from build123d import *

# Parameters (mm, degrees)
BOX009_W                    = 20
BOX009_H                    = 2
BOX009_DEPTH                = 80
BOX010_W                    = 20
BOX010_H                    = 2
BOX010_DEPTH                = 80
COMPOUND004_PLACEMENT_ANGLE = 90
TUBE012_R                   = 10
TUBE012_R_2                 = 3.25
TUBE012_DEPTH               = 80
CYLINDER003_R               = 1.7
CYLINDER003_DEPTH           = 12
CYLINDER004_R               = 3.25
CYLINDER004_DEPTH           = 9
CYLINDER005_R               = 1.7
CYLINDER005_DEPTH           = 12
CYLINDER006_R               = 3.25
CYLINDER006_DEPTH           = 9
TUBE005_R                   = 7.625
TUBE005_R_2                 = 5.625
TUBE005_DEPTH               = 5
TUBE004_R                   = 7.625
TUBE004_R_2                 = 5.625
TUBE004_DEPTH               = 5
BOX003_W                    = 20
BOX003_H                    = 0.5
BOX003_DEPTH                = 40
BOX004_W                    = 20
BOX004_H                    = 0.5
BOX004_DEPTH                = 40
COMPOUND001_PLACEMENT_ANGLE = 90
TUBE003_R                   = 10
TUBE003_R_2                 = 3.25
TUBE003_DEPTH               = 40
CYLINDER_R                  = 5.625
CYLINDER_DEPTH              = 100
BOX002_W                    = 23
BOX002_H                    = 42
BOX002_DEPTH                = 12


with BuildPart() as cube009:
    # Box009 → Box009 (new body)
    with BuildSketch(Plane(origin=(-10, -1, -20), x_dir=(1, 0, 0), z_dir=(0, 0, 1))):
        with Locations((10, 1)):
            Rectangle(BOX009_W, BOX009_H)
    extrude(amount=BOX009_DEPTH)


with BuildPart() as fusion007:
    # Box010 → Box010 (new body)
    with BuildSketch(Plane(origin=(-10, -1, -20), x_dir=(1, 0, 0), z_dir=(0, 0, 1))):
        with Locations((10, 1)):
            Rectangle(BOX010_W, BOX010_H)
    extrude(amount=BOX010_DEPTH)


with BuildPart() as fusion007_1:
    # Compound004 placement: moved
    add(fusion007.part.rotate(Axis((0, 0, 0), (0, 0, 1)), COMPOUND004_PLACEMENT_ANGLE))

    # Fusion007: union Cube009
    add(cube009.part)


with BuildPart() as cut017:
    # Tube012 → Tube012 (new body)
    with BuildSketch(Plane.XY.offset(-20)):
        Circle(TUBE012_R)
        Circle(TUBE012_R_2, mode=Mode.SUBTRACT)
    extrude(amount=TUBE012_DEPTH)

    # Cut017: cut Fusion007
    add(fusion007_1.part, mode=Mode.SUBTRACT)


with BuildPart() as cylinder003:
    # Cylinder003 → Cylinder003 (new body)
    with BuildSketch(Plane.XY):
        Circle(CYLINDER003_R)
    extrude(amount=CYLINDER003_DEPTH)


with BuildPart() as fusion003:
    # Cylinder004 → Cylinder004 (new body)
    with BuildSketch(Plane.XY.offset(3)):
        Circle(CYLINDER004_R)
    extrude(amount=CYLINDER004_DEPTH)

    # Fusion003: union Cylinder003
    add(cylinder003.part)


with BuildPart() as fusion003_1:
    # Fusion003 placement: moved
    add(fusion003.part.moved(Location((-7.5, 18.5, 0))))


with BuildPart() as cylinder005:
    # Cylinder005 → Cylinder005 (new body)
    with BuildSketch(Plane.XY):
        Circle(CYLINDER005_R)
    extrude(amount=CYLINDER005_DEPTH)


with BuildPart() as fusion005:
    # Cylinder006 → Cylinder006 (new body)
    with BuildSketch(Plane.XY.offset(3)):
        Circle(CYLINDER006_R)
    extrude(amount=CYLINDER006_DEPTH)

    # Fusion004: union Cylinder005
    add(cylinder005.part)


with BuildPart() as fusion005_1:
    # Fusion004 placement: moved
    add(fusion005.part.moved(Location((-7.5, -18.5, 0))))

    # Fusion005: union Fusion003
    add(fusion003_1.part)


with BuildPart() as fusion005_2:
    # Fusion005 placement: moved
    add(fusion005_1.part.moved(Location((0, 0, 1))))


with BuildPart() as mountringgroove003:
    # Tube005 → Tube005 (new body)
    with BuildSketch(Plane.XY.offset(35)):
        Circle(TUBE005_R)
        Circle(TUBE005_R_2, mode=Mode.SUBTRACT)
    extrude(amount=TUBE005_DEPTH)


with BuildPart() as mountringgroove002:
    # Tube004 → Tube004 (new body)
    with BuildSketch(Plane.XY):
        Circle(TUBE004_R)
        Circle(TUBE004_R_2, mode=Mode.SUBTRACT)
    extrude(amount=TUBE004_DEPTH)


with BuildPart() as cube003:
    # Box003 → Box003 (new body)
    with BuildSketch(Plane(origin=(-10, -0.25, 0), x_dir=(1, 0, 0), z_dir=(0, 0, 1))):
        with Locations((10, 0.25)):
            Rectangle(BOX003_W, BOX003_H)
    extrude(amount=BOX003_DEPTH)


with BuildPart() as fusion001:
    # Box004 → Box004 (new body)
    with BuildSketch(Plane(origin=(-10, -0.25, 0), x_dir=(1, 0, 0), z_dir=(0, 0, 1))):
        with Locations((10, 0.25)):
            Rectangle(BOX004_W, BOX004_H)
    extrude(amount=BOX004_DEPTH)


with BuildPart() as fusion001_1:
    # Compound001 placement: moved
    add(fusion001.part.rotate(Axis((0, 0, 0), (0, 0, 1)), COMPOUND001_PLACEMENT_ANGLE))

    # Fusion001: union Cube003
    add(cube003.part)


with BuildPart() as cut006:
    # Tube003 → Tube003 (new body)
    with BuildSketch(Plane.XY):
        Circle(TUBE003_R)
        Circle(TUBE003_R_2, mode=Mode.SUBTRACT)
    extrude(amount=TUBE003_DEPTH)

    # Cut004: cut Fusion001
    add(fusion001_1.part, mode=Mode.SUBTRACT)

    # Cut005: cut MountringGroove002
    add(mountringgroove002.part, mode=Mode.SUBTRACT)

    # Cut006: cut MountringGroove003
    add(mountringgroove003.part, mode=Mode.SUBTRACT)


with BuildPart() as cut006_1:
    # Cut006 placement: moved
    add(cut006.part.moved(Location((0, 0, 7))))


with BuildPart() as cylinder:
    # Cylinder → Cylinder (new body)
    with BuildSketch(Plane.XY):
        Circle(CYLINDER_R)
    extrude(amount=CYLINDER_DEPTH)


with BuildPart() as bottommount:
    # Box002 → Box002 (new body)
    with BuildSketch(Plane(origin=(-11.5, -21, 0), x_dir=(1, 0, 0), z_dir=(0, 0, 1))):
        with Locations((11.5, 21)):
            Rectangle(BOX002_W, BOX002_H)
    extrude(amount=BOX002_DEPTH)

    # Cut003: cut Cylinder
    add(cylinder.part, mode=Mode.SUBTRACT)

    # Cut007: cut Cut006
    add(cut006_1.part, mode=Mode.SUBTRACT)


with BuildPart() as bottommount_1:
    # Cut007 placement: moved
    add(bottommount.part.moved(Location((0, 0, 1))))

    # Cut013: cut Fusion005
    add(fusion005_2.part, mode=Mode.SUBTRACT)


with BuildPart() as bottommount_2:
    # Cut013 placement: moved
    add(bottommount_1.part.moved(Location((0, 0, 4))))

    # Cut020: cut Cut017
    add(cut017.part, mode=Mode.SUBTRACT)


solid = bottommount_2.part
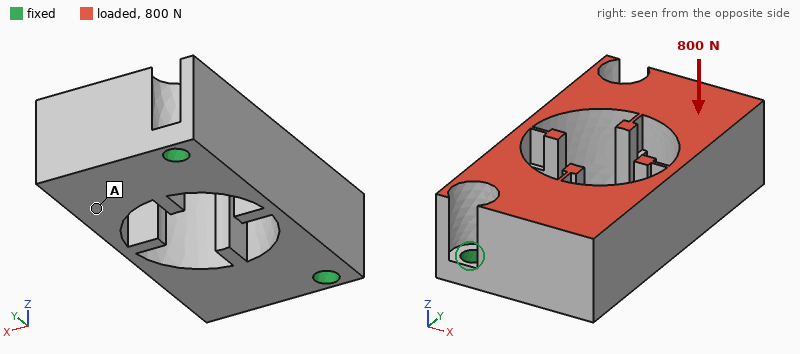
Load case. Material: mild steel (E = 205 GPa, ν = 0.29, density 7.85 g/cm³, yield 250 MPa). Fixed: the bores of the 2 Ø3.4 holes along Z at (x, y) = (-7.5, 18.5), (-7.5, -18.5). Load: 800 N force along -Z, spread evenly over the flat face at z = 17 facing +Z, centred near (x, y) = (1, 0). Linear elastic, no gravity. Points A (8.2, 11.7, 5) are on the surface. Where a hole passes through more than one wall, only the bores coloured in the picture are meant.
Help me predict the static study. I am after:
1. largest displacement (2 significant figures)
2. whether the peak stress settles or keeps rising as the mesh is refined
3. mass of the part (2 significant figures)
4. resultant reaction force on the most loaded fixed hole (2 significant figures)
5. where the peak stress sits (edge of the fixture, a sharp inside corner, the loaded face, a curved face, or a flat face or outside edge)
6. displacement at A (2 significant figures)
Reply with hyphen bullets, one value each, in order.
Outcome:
- 22 µm
- keeps rising
- 59 g
- 420 N
- edge of the fixture
- 15 µm
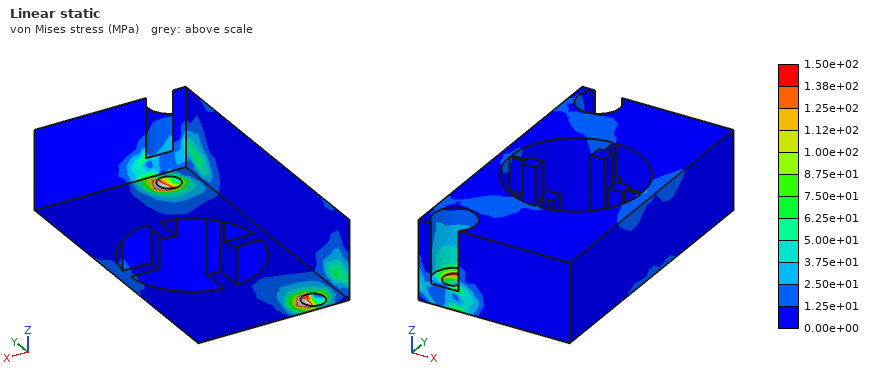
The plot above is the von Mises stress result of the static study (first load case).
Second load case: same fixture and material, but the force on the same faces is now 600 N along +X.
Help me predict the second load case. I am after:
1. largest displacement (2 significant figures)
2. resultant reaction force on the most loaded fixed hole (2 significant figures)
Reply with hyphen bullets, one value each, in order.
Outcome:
- 20 µm
- 300 N
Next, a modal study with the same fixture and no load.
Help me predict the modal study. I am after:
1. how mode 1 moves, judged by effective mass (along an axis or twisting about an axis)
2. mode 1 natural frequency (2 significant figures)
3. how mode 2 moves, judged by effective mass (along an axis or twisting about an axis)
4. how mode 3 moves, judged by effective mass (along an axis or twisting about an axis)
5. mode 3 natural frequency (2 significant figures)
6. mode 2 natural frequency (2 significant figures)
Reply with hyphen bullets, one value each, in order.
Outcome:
- along Z
- 4600 Hz
- along Y
- twisting about X
- 12 kHz
- 9900 Hz
